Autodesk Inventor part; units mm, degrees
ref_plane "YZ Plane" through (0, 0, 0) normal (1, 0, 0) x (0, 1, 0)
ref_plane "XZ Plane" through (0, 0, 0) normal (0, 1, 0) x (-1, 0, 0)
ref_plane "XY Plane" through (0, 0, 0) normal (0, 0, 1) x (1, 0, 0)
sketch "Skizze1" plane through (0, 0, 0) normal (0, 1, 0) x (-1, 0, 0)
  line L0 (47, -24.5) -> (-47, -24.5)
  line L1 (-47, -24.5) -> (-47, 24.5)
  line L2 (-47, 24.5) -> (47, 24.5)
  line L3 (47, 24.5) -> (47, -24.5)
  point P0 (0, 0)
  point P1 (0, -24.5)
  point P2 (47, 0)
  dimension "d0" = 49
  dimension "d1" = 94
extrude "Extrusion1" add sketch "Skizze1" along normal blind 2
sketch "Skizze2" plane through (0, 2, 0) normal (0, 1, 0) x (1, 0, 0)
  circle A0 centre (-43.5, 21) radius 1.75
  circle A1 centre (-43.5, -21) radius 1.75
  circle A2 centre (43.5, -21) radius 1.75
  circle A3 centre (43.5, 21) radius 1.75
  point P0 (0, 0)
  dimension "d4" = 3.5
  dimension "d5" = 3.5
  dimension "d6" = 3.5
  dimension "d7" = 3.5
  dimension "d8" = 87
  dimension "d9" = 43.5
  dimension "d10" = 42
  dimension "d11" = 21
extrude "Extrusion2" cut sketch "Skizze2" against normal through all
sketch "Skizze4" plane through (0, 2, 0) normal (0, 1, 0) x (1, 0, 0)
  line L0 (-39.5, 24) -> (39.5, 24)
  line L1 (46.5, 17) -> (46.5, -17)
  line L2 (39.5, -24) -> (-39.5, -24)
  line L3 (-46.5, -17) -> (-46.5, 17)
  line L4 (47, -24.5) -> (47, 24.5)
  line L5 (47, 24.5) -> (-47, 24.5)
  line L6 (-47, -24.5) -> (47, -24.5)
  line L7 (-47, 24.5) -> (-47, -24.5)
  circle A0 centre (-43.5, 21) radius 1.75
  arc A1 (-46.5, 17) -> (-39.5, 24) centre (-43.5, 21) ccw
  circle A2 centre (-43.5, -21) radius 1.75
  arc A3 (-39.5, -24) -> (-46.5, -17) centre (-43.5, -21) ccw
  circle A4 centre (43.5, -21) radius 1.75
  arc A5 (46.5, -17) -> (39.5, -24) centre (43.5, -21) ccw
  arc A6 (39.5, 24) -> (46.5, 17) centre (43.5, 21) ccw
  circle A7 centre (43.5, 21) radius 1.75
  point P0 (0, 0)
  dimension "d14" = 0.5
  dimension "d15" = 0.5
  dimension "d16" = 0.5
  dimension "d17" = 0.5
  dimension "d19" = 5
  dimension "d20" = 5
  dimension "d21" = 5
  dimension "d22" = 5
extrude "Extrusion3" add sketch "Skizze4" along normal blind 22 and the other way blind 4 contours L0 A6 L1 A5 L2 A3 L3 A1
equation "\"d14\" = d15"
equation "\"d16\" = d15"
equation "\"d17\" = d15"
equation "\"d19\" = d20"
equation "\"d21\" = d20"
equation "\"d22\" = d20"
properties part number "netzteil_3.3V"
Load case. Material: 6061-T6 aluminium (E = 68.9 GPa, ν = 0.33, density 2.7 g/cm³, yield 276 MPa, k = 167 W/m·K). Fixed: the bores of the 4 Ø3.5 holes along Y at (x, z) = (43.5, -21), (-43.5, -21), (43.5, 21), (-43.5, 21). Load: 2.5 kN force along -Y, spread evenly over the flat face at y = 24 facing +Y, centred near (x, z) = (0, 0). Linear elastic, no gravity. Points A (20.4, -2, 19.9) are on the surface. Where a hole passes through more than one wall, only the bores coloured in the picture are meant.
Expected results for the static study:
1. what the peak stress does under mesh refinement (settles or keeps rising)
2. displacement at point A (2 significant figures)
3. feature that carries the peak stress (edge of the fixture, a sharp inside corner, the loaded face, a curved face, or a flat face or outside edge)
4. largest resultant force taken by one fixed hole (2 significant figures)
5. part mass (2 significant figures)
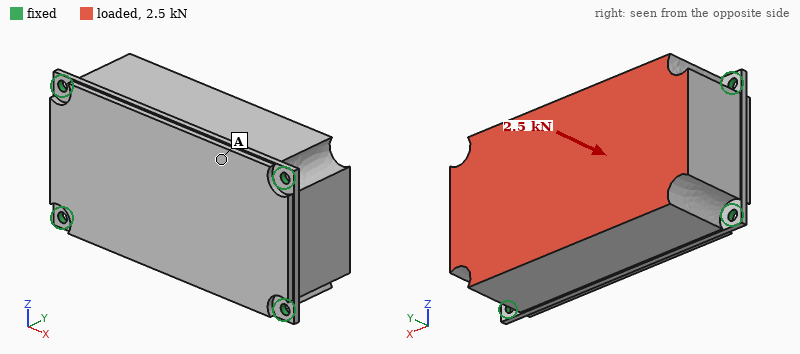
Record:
keeps rising
13 µm
edge of the fixture
670 N
300 g
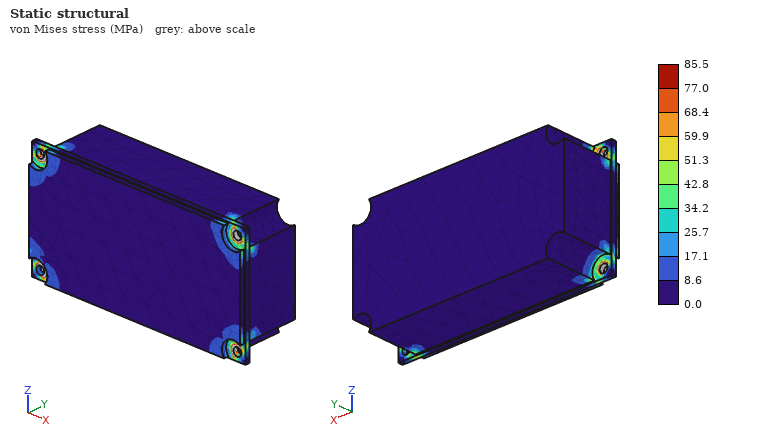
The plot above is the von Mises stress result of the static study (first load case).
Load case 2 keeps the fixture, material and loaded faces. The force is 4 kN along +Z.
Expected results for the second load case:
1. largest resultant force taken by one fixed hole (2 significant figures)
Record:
1.6 kN
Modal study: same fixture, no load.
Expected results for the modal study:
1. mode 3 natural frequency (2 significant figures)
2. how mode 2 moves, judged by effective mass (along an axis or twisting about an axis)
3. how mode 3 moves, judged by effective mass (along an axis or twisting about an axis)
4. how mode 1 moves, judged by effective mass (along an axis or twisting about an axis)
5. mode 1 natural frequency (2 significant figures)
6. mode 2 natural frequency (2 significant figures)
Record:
6100 Hz
along Z
along X
along Y
4000 Hz
4400 Hz
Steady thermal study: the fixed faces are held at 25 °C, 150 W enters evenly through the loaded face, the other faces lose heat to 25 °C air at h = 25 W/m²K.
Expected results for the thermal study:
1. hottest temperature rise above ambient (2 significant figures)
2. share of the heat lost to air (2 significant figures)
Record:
52 K
9.1 %
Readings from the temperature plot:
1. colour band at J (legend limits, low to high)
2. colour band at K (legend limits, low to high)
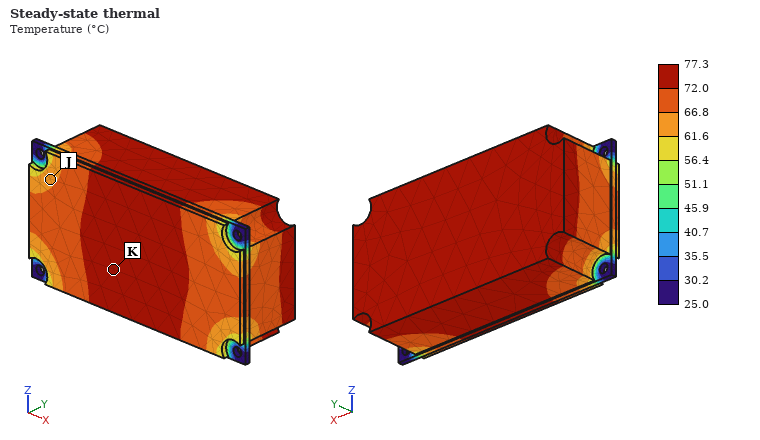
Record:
61.6 to 66.8 °C
72.0 to 77.3 °C
